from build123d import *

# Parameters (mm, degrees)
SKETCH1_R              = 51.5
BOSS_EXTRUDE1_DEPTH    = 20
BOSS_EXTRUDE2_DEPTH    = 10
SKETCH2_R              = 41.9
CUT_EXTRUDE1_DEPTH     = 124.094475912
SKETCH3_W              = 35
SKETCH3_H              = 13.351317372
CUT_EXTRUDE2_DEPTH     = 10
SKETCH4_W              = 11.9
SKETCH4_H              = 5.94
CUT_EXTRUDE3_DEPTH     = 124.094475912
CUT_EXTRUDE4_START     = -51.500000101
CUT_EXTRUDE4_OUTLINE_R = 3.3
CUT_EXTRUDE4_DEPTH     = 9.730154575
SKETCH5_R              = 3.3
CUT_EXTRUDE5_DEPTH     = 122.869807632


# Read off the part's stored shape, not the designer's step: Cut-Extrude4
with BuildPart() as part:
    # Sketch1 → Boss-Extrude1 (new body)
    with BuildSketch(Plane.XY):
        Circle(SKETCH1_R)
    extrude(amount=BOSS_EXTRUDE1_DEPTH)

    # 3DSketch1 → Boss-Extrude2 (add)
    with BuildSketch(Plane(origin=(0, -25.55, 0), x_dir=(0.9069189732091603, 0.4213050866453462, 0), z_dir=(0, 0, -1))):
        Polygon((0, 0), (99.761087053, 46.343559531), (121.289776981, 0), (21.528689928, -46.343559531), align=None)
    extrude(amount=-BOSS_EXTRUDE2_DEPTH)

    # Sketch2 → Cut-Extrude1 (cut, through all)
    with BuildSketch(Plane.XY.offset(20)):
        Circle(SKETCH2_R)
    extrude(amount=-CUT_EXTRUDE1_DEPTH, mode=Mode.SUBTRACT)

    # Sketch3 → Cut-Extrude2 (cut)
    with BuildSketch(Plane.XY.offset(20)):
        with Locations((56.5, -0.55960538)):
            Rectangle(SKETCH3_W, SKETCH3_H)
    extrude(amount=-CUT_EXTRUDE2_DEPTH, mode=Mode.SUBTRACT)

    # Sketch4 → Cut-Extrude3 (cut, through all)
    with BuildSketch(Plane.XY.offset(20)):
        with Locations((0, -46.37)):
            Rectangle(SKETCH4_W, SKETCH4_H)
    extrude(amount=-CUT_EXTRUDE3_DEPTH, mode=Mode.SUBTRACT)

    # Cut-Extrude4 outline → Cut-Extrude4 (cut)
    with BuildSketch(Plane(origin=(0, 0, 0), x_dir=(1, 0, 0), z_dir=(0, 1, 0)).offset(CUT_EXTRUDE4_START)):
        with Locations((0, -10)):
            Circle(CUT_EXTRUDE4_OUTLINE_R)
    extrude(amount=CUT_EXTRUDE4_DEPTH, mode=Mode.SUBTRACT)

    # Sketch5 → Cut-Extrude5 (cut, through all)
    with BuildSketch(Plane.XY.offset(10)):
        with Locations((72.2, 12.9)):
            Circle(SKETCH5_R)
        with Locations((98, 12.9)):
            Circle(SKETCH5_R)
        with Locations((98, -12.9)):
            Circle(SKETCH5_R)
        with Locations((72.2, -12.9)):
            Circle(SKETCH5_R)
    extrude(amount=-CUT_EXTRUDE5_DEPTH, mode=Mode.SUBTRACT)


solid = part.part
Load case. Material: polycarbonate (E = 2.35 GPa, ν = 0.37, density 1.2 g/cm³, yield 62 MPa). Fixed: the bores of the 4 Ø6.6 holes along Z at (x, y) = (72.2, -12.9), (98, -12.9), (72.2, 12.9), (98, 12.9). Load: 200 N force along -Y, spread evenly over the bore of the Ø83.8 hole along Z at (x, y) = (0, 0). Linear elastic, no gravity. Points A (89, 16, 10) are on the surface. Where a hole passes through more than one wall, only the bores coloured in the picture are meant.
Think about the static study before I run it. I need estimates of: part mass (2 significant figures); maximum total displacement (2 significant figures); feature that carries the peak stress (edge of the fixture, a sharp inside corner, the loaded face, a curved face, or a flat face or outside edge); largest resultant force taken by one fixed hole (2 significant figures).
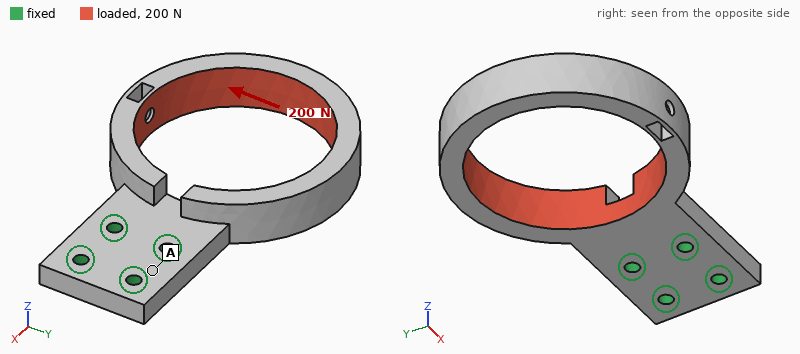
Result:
100 g
2.0 mm
the loaded face
390 N
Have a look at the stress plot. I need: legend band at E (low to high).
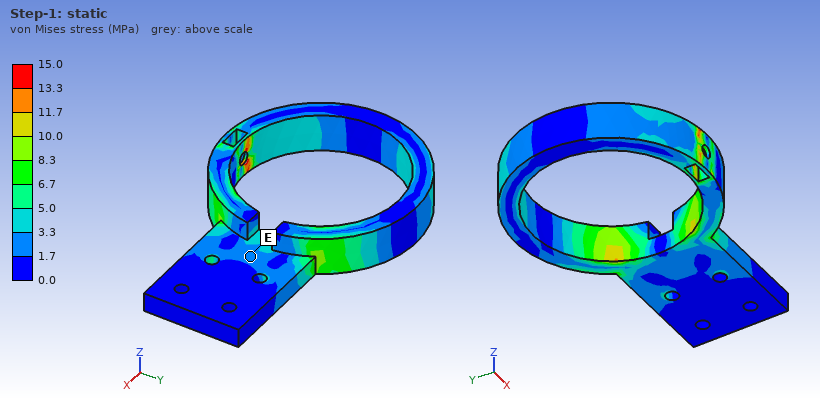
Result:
1.7 to 3.3 MPa
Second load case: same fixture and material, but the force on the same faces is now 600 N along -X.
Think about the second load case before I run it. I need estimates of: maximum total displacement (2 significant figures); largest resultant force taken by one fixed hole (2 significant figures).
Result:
1.4 mm
280 N
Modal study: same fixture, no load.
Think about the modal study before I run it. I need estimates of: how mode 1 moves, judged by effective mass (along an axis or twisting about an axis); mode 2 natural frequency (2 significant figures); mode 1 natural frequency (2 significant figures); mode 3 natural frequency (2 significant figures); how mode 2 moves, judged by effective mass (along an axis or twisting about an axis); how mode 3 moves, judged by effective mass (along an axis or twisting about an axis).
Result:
along Z
220 Hz
140 Hz
340 Hz
along Y
twisting about X
